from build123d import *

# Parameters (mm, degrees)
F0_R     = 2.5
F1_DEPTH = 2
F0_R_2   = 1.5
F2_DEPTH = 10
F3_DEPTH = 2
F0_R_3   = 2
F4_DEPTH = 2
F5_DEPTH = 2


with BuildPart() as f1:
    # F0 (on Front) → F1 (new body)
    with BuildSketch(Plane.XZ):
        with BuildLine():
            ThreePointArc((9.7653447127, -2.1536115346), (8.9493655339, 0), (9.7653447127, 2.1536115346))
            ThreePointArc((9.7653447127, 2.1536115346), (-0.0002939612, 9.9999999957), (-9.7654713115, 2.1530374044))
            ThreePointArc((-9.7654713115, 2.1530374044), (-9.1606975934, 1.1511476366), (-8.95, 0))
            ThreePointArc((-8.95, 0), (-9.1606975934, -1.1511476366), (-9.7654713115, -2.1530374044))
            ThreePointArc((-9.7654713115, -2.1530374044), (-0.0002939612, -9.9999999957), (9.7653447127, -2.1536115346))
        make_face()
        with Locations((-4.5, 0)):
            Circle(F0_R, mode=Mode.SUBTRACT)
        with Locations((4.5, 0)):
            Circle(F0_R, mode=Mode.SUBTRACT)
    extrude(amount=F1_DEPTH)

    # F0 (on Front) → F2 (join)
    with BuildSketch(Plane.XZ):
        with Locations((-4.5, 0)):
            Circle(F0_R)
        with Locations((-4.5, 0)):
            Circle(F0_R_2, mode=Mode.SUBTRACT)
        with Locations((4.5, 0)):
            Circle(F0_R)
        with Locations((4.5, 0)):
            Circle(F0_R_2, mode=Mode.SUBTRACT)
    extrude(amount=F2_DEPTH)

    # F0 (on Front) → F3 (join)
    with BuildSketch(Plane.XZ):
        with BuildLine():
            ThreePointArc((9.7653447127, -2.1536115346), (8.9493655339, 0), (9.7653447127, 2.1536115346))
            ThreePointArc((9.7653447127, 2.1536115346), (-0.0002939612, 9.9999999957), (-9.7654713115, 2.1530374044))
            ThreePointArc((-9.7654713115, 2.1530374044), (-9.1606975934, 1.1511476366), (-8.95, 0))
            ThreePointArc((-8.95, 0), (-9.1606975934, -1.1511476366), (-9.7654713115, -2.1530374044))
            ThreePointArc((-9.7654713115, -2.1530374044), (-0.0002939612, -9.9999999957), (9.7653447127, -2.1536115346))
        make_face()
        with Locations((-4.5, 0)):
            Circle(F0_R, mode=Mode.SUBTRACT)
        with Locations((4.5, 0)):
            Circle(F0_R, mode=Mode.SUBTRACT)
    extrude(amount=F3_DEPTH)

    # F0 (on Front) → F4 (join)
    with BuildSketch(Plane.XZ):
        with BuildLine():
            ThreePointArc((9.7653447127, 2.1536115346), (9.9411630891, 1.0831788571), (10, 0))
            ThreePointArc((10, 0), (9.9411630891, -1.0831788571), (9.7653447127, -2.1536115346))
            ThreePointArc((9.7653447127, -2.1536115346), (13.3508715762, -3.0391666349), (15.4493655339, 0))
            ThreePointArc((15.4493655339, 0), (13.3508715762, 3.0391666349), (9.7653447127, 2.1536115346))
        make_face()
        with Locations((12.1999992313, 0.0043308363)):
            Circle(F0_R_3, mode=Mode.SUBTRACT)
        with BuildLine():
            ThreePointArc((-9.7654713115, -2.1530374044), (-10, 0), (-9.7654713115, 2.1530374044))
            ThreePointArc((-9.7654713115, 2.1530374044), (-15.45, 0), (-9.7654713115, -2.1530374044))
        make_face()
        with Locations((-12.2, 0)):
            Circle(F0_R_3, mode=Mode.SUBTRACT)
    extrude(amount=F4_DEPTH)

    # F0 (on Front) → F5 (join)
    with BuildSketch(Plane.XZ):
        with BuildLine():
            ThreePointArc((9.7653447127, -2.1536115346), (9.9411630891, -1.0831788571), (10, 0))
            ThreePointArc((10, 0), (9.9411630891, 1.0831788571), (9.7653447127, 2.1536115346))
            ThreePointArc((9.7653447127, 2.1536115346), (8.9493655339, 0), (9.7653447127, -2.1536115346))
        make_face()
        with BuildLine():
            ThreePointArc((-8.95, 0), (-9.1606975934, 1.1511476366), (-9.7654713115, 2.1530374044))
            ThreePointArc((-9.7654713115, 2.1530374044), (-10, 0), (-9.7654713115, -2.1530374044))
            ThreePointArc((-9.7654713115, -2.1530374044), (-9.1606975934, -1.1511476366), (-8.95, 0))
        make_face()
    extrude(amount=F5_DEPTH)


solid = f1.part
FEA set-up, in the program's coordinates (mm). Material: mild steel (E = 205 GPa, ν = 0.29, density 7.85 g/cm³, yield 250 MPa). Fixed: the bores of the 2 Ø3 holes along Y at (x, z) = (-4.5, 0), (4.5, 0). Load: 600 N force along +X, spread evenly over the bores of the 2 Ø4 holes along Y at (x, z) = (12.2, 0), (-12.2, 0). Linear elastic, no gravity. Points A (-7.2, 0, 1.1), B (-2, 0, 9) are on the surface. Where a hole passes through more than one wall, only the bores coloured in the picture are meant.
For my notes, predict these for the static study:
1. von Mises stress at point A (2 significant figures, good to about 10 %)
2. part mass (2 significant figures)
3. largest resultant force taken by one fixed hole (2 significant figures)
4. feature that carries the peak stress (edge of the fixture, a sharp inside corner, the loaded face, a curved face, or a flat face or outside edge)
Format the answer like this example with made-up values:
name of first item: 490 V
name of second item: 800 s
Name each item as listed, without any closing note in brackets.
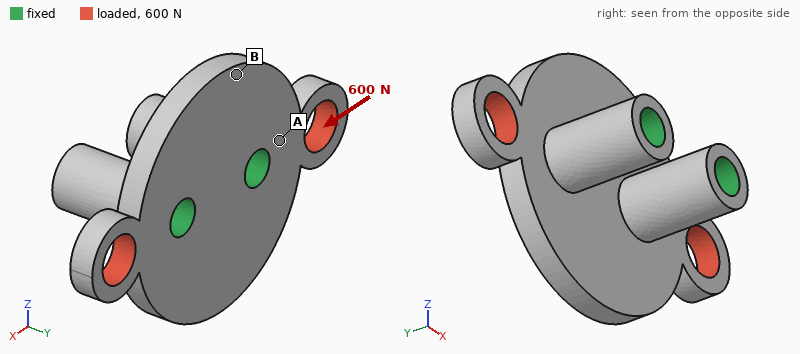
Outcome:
von Mises stress at point A: 26 MPa
part mass: 6.8 g
largest resultant force taken by one fixed hole: 300 N
feature that carries the peak stress: the loaded face
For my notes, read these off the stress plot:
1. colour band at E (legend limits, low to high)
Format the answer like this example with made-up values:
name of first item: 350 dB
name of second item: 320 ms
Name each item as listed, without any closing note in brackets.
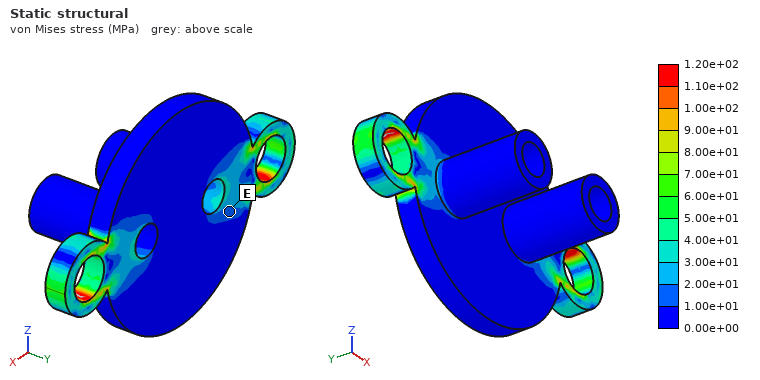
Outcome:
colour band at E: 1.00e+01 to 2.00e+01 MPa
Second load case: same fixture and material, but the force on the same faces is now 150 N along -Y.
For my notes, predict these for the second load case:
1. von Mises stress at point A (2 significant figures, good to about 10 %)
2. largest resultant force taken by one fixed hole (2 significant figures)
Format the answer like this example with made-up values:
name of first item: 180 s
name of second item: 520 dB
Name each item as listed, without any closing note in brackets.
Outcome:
von Mises stress at point A: 66 MPa
largest resultant force taken by one fixed hole: 76 N
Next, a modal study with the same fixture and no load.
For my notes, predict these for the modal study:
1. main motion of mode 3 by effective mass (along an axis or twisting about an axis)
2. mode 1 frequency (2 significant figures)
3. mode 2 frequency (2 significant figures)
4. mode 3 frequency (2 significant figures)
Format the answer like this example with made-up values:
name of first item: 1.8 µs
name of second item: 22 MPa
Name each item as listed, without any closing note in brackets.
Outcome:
main motion of mode 3 by effective mass: twisting about X
mode 1 frequency: 22 kHz
mode 2 frequency: 23 kHz
mode 3 frequency: 26 kHz
